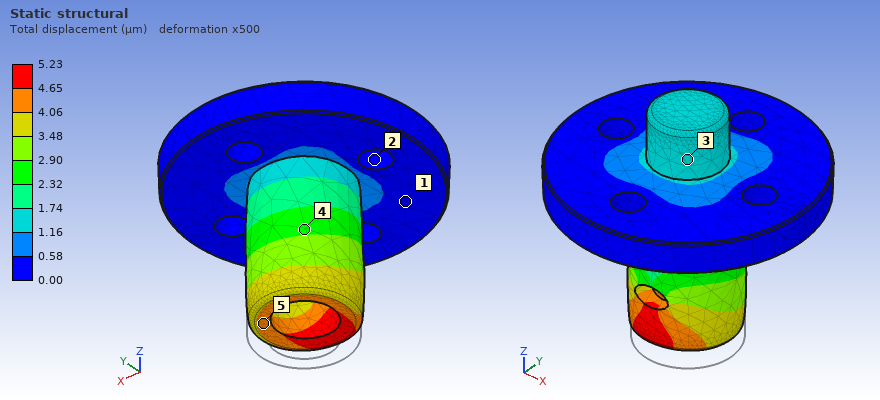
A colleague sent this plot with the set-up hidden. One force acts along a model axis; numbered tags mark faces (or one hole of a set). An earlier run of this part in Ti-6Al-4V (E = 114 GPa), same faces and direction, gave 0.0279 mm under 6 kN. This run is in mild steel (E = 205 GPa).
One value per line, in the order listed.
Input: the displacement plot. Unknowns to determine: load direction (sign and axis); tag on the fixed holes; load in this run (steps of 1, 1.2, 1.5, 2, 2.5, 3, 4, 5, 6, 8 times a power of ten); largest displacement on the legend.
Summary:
+Z
2
2 kN
5.23 µm
